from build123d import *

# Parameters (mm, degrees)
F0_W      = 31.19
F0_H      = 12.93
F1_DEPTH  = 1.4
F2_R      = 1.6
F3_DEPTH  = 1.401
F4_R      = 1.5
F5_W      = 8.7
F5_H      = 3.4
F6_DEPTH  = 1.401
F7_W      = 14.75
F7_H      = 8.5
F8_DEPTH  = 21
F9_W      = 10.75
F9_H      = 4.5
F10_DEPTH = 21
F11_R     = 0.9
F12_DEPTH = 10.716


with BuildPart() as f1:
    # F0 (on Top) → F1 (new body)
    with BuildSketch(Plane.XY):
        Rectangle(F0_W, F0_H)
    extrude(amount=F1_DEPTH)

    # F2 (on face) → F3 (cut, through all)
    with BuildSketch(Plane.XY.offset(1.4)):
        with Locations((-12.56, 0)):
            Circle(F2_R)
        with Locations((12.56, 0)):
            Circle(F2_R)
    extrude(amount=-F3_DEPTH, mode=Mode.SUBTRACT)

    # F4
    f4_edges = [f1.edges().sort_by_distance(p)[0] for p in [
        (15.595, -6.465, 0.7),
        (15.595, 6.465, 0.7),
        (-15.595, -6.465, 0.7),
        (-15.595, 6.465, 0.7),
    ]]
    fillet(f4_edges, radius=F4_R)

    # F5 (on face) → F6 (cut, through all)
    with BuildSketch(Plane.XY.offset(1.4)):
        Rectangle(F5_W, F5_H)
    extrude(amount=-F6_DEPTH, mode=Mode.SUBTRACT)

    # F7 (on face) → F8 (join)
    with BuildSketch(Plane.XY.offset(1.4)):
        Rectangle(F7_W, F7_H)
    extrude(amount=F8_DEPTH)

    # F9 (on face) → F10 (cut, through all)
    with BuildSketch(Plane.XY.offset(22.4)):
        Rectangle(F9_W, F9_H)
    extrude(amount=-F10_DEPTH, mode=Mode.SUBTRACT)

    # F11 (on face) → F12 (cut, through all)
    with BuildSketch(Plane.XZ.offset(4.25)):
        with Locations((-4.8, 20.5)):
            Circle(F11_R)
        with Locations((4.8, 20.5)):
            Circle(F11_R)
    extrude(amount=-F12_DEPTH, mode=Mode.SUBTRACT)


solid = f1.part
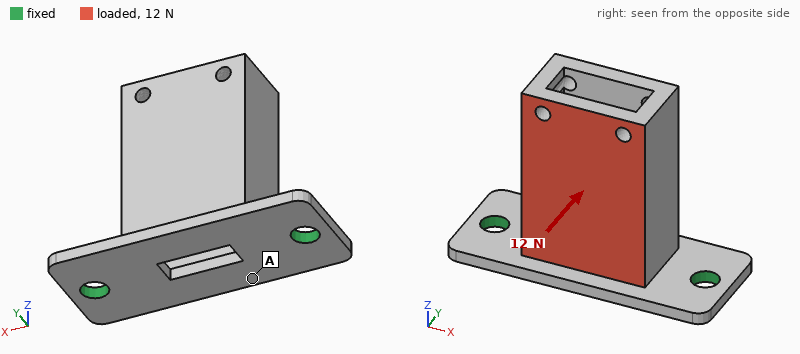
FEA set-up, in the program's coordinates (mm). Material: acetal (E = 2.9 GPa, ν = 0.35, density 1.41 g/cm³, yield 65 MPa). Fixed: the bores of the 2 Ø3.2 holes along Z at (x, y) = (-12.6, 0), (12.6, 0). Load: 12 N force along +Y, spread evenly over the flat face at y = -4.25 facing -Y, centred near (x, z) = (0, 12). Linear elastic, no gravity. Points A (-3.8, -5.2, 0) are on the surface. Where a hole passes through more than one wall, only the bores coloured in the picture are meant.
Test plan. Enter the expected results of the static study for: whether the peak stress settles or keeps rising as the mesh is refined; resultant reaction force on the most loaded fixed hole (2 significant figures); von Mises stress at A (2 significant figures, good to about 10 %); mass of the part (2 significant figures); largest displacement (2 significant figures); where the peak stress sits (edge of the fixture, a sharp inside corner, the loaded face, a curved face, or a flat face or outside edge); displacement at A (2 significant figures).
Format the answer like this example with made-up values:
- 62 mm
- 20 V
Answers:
- keeps rising
- 6.0 N
- 2.2 MPa
- 2.9 g
- 0.39 mm
- edge of the fixture
- 0.090 mm
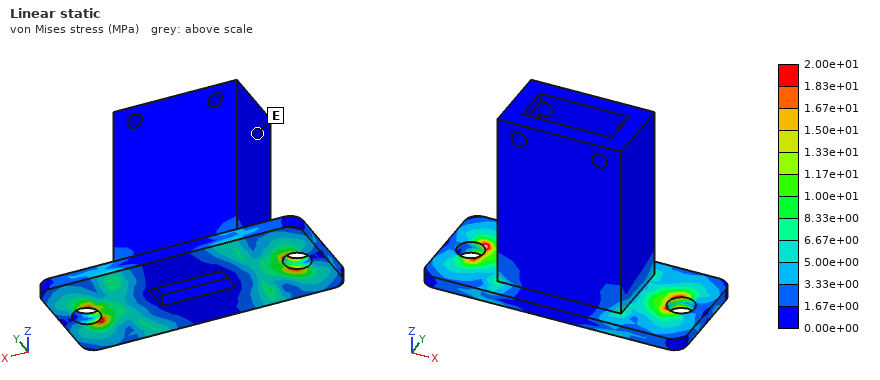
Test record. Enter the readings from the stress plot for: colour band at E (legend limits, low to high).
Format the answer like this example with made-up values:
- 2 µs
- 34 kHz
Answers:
- 0.00e+00 to 1.67e+00 MPa
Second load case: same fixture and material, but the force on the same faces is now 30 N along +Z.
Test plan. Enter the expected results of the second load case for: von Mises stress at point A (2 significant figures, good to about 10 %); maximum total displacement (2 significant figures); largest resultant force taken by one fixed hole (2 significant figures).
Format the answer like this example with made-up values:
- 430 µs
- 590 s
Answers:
- 2.5 MPa
- 0.38 mm
- 17 N
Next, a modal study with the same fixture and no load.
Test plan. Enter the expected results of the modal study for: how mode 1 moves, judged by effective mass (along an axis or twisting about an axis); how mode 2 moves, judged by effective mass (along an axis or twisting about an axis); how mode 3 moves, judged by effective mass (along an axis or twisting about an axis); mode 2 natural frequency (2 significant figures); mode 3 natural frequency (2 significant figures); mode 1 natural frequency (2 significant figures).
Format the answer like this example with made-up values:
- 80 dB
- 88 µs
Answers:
- along Y
- along X
- along Z
- 2200 Hz
- 3000 Hz
- 710 Hz
